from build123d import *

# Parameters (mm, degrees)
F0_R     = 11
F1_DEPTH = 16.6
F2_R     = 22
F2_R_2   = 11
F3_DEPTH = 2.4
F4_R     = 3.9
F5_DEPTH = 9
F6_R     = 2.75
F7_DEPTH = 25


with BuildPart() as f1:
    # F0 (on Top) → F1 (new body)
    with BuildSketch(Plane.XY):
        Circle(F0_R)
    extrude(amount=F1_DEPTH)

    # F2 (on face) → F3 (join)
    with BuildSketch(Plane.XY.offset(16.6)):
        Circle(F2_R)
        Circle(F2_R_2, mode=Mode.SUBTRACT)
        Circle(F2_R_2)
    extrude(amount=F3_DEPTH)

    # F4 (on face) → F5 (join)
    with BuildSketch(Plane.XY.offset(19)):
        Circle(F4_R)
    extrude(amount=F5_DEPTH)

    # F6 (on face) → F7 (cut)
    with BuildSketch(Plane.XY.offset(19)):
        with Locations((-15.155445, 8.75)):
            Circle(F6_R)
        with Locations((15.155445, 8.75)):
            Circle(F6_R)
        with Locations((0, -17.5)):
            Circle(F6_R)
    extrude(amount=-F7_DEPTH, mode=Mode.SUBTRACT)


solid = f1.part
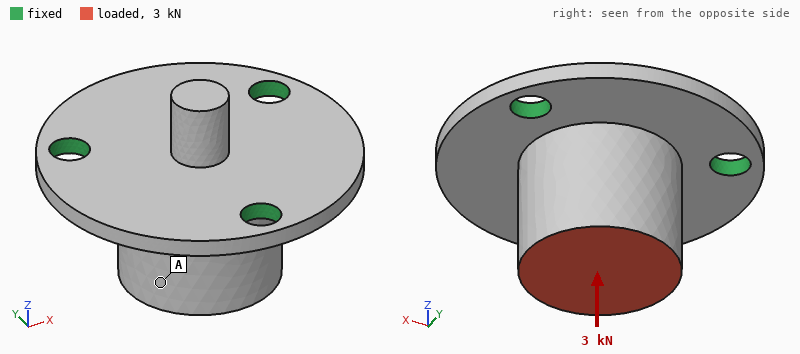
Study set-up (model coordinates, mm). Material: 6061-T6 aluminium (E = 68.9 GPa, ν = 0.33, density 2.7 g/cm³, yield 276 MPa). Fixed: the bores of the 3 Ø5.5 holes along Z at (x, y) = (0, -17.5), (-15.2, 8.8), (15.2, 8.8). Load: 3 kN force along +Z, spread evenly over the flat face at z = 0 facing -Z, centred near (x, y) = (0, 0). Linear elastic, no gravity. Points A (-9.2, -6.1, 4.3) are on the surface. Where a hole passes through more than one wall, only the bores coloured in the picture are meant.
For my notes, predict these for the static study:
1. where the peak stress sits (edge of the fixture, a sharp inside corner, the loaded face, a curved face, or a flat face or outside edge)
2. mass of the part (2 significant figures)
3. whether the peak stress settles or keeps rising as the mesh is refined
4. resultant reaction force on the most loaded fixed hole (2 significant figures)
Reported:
edge of the fixture
28 g
keeps rising
1.1 kN
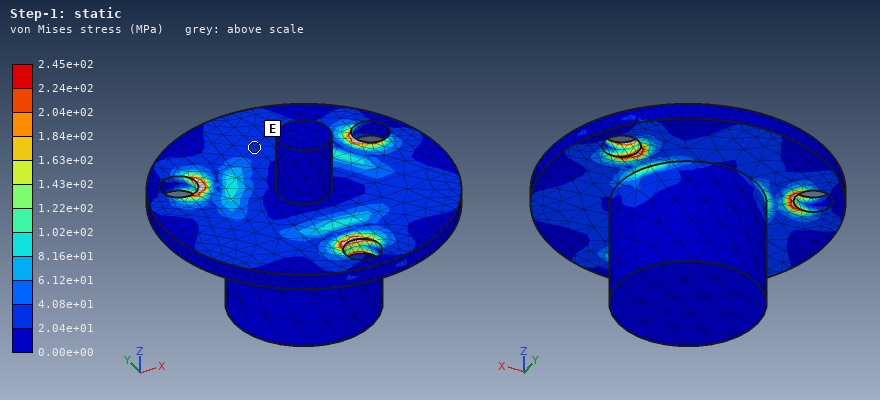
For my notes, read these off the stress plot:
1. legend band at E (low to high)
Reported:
2.04e+01 to 4.08e+01 MPa
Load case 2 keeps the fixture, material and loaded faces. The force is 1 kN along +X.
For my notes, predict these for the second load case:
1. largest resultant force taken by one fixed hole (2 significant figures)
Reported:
830 N
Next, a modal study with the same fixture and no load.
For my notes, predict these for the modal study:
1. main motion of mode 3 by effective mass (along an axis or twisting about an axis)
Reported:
along Z
